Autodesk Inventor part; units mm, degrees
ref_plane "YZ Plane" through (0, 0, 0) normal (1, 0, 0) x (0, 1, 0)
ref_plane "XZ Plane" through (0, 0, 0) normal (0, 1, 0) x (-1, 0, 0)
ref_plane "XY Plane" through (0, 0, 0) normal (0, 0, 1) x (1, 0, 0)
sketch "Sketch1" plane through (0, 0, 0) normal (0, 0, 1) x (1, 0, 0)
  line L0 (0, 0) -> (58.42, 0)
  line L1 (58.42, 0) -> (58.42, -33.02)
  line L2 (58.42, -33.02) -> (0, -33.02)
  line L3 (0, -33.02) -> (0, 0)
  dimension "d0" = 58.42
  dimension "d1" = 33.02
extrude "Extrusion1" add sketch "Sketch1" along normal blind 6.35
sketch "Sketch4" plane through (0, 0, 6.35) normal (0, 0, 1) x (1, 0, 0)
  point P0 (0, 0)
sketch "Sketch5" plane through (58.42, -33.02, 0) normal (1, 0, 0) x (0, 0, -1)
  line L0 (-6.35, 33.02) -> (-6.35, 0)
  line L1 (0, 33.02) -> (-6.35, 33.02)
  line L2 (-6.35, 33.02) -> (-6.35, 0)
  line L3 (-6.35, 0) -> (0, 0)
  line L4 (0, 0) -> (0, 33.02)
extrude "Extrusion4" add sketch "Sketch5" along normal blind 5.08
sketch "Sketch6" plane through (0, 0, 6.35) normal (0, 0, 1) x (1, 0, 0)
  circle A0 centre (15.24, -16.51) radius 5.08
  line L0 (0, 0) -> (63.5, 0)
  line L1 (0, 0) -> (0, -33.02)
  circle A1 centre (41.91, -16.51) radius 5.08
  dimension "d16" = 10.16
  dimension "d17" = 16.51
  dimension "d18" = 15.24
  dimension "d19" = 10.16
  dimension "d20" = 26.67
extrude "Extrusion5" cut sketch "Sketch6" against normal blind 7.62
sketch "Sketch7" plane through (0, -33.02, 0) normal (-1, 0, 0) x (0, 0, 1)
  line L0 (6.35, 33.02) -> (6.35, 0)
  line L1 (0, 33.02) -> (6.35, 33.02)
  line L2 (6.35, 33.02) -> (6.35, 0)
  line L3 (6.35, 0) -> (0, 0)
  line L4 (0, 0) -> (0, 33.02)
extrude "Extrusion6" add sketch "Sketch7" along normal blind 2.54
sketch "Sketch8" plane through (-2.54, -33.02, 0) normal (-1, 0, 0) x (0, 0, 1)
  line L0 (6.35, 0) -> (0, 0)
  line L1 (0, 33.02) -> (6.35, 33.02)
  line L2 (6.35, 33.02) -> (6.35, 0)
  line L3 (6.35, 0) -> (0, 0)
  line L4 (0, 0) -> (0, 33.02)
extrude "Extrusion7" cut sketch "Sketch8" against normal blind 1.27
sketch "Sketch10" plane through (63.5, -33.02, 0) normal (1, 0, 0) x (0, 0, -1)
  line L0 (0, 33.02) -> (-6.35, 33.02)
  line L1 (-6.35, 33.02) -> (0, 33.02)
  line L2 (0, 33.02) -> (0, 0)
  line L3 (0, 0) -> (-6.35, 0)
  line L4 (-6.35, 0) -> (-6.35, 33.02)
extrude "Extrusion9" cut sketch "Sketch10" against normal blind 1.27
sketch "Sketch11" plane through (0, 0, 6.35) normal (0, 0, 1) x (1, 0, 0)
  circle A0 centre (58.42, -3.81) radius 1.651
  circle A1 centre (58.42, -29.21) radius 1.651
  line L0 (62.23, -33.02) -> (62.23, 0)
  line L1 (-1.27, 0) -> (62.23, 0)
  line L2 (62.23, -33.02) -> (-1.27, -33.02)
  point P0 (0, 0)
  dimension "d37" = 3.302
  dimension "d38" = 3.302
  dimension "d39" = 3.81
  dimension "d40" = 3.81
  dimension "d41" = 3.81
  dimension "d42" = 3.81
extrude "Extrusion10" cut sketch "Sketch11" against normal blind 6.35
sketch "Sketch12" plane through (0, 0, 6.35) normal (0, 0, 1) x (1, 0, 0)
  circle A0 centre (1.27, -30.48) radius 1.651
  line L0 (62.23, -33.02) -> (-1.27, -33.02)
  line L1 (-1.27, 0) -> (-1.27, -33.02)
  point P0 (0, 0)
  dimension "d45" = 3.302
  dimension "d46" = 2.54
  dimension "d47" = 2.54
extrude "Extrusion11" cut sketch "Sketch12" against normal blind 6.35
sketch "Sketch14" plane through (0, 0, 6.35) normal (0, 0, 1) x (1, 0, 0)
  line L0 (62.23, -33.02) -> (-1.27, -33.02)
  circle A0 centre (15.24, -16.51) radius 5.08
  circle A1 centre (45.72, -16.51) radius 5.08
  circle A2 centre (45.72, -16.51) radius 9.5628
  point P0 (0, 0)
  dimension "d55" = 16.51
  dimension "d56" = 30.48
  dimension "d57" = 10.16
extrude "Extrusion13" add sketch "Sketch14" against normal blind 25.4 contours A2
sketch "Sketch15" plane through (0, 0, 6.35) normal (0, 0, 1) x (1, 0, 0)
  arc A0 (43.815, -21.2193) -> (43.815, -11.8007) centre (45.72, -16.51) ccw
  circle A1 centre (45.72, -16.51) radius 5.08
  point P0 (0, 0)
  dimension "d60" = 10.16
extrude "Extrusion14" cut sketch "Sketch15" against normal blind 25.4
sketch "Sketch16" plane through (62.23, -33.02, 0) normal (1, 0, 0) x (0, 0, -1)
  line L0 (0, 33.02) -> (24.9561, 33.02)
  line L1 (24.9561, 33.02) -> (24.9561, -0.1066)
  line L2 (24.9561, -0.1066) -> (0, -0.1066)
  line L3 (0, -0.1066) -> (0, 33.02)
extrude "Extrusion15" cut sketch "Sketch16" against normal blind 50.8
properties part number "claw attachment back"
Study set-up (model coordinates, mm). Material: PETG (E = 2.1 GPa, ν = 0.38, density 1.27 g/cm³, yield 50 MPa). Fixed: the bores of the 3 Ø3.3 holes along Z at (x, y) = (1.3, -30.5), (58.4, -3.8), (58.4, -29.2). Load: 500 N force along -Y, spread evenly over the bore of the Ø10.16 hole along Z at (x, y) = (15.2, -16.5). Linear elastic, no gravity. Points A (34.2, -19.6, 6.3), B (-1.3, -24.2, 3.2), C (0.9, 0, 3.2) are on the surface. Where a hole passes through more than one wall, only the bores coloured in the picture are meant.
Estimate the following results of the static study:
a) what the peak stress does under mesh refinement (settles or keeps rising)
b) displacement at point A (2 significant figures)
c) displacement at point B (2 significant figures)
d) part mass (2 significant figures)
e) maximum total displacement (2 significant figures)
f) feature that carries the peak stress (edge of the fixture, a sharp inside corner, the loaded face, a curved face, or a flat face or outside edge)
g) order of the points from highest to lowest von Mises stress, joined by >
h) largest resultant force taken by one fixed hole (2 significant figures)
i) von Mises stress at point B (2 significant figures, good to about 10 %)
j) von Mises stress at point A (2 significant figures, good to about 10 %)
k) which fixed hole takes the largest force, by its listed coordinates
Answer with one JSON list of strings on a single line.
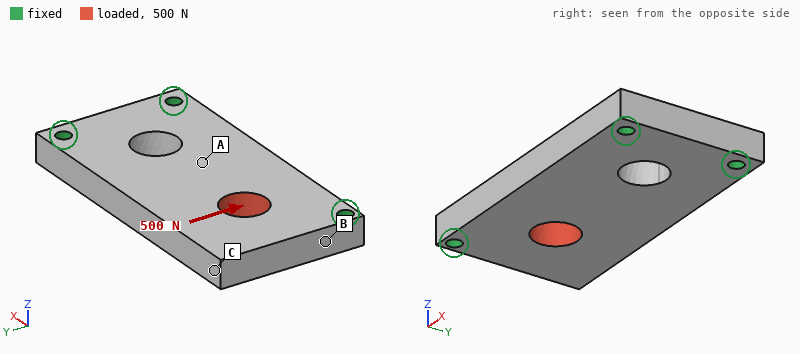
["keeps rising", "56 µm", "13 µm", "15 g", "82 µm", "edge of the fixture", "B > A > C", "360 N", "6.2 MPa", "2.4 MPa", "(1.3, -30.5)"]
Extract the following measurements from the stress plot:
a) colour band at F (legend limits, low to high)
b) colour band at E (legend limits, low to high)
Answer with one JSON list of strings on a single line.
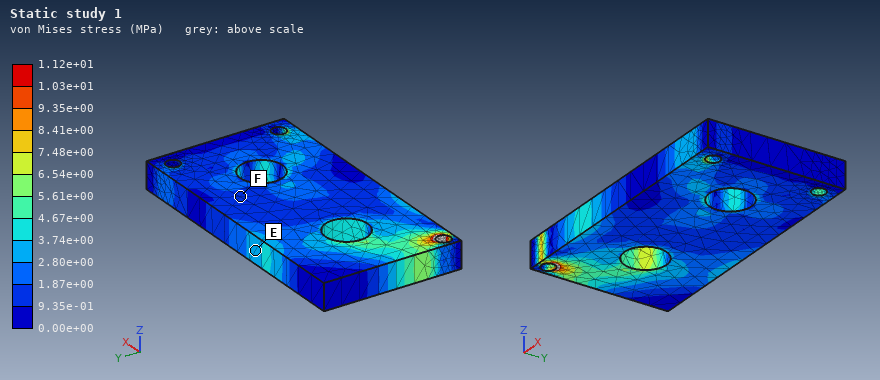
["9.35e-01 to 1.87e+00 MPa", "2.80e+00 to 3.74e+00 MPa"]
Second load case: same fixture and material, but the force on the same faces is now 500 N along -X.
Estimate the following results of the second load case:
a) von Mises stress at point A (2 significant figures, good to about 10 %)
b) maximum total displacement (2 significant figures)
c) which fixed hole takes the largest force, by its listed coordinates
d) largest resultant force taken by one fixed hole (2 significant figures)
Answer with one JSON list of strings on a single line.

["1.9 MPa", "57 µm", "(1.3, -30.5)", "210 N"]
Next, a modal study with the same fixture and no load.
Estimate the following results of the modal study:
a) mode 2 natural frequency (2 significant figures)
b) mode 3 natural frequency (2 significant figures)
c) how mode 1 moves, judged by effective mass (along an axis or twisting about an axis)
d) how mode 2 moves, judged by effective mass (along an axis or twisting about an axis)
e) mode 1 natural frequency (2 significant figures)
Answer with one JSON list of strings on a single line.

["2300 Hz", "3500 Hz", "along Z", "along Z", "1200 Hz"]
